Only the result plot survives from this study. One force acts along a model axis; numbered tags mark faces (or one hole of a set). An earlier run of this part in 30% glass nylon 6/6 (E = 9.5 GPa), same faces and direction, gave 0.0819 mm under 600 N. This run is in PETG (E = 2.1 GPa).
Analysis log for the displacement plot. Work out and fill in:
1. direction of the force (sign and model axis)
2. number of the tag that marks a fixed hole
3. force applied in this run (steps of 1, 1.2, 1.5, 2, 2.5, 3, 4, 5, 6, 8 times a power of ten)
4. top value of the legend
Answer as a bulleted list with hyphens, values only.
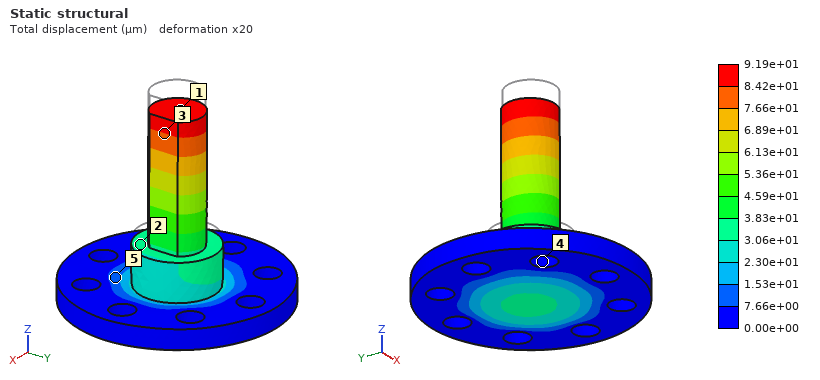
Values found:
- -Z
- 4
- 150 N
- 9.19e+01 µm
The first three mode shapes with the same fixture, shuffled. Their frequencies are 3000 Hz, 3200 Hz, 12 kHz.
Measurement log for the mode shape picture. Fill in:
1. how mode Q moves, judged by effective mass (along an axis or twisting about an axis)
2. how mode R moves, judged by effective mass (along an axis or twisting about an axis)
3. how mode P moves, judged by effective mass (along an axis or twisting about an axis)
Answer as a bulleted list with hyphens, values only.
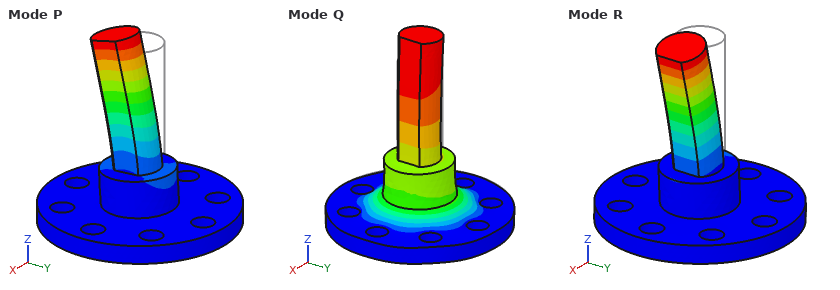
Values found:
- along Z
- along X
- along Y
